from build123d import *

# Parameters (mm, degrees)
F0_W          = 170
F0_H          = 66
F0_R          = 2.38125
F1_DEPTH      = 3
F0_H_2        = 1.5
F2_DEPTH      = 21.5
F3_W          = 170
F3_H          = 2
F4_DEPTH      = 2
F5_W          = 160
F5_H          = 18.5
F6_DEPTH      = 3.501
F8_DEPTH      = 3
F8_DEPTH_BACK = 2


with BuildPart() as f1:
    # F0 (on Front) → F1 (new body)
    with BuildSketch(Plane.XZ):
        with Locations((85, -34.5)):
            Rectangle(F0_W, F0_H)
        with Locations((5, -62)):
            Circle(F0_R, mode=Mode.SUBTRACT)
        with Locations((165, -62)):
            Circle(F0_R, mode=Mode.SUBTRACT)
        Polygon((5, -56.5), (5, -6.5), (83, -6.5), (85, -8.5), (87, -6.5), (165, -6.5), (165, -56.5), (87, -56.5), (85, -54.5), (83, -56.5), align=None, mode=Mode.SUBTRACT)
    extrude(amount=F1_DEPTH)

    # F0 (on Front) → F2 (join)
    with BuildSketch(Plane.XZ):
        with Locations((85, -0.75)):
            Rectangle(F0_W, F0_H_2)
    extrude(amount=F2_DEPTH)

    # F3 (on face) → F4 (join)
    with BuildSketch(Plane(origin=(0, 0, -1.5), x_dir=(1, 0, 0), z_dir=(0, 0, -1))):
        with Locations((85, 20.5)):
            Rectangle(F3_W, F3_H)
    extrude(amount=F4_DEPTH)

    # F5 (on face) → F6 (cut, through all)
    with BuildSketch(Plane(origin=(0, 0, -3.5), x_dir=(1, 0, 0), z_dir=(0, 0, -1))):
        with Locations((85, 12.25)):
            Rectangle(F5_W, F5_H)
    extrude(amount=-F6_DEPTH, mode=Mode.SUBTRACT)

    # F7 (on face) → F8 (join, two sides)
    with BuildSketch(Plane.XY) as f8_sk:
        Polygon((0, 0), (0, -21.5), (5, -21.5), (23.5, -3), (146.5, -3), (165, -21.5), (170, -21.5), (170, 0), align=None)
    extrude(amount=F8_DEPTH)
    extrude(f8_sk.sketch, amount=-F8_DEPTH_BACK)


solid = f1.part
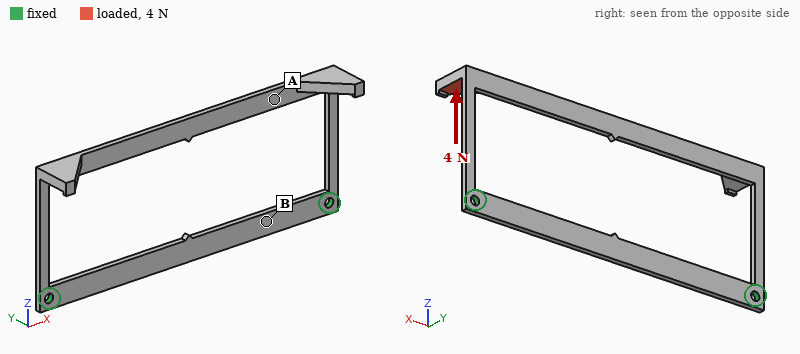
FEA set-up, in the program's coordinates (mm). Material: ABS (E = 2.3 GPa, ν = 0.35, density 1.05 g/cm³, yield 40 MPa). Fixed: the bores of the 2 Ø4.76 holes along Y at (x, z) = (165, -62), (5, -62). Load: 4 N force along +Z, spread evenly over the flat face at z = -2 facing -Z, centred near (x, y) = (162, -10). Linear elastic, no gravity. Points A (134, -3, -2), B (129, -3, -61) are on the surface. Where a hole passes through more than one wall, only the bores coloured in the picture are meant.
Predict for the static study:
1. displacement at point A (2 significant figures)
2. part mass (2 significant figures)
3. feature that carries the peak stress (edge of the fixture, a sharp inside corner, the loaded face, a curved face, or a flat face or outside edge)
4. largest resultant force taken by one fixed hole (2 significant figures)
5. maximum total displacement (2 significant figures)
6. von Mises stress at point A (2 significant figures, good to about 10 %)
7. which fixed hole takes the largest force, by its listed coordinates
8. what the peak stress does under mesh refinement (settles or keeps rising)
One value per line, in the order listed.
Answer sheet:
1.3 mm
15 g
a sharp inside corner
3.9 N
1.9 mm
0.81 MPa
(165, -62)
keeps rising
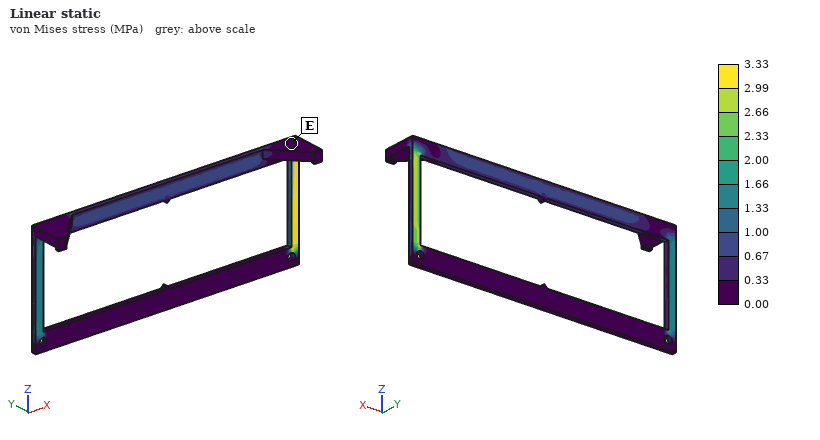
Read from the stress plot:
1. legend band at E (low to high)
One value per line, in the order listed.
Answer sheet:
0.00 to 0.33 MPa
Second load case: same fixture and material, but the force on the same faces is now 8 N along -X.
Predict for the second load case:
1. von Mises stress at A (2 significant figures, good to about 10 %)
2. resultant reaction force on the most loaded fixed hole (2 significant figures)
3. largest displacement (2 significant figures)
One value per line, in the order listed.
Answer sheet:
2.8 MPa
4.3 N
1.9 mm
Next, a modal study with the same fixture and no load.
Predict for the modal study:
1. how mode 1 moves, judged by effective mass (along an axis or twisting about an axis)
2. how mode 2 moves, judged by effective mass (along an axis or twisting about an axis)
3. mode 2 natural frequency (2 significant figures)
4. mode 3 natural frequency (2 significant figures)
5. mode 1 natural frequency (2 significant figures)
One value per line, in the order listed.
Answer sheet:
along Y
twisting about Z
91 Hz
140 Hz
45 Hz
